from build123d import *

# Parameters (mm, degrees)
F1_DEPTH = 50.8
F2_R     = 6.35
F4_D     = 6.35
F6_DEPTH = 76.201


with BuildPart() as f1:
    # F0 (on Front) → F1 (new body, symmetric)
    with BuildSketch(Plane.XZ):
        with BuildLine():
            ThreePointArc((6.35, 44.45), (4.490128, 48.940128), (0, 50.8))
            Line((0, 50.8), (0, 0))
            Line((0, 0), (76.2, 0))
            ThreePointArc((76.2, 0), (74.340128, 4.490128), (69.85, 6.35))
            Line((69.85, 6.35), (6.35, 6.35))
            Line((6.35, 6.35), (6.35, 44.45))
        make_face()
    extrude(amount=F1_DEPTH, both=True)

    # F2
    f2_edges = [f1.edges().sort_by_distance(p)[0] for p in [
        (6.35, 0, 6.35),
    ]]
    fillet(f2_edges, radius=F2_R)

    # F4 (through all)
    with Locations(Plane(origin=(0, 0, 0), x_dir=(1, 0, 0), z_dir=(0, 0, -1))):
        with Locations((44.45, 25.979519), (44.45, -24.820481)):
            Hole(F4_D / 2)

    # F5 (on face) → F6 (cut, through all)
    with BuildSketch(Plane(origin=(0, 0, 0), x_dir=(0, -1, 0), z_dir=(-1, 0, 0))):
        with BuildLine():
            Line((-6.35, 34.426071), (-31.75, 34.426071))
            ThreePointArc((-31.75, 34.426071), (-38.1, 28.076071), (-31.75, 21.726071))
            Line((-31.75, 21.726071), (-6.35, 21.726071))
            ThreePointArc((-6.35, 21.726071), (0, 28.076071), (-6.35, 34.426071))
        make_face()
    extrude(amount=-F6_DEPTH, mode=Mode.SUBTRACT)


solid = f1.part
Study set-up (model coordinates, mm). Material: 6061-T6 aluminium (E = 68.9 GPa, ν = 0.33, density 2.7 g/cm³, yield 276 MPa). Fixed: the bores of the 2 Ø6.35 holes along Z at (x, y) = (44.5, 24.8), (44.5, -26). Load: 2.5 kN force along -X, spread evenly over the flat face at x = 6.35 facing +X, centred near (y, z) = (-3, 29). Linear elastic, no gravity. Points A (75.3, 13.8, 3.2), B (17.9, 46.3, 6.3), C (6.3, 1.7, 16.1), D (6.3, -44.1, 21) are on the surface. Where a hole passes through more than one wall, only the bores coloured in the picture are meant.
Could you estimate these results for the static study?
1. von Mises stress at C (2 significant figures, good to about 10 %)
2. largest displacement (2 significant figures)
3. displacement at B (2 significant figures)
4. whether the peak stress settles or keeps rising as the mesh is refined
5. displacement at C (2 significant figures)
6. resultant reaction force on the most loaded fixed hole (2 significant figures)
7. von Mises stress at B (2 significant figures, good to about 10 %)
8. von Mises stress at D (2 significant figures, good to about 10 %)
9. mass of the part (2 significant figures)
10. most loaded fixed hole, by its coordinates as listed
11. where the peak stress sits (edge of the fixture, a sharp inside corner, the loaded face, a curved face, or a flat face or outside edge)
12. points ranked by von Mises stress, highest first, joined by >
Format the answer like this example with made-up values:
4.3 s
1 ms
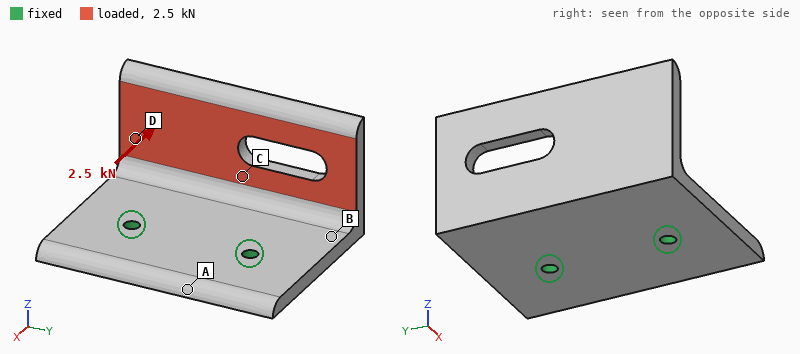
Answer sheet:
61 MPa
1.1 mm
0.16 mm
keeps rising
0.39 mm
1.4 kN
87 MPa
34 MPa
200 g
(44.5, -26)
edge of the fixture
B > C > D > A
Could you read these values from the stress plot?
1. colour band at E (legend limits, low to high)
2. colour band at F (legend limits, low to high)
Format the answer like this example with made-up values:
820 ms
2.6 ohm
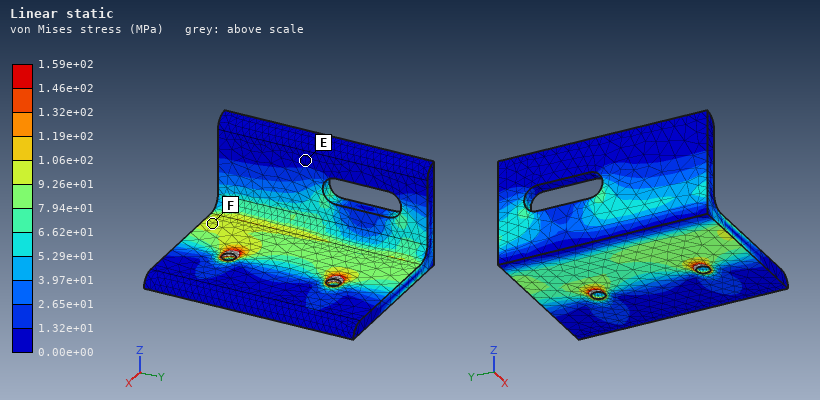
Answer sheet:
0.00e+00 to 1.32e+01 MPa
9.26e+01 to 1.06e+02 MPa
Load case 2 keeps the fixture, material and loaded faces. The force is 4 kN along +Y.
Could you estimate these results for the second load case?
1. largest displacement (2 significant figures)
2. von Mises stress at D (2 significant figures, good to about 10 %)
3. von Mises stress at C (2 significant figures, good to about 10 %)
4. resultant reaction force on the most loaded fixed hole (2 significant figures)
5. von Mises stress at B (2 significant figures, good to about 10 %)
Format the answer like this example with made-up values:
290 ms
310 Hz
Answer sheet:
0.60 mm
44 MPa
66 MPa
3.8 kN
46 MPa
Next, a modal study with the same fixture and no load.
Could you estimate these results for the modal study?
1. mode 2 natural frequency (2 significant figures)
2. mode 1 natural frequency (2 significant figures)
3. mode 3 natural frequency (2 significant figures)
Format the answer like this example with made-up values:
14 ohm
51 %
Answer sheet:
1500 Hz
910 Hz
2500 Hz
